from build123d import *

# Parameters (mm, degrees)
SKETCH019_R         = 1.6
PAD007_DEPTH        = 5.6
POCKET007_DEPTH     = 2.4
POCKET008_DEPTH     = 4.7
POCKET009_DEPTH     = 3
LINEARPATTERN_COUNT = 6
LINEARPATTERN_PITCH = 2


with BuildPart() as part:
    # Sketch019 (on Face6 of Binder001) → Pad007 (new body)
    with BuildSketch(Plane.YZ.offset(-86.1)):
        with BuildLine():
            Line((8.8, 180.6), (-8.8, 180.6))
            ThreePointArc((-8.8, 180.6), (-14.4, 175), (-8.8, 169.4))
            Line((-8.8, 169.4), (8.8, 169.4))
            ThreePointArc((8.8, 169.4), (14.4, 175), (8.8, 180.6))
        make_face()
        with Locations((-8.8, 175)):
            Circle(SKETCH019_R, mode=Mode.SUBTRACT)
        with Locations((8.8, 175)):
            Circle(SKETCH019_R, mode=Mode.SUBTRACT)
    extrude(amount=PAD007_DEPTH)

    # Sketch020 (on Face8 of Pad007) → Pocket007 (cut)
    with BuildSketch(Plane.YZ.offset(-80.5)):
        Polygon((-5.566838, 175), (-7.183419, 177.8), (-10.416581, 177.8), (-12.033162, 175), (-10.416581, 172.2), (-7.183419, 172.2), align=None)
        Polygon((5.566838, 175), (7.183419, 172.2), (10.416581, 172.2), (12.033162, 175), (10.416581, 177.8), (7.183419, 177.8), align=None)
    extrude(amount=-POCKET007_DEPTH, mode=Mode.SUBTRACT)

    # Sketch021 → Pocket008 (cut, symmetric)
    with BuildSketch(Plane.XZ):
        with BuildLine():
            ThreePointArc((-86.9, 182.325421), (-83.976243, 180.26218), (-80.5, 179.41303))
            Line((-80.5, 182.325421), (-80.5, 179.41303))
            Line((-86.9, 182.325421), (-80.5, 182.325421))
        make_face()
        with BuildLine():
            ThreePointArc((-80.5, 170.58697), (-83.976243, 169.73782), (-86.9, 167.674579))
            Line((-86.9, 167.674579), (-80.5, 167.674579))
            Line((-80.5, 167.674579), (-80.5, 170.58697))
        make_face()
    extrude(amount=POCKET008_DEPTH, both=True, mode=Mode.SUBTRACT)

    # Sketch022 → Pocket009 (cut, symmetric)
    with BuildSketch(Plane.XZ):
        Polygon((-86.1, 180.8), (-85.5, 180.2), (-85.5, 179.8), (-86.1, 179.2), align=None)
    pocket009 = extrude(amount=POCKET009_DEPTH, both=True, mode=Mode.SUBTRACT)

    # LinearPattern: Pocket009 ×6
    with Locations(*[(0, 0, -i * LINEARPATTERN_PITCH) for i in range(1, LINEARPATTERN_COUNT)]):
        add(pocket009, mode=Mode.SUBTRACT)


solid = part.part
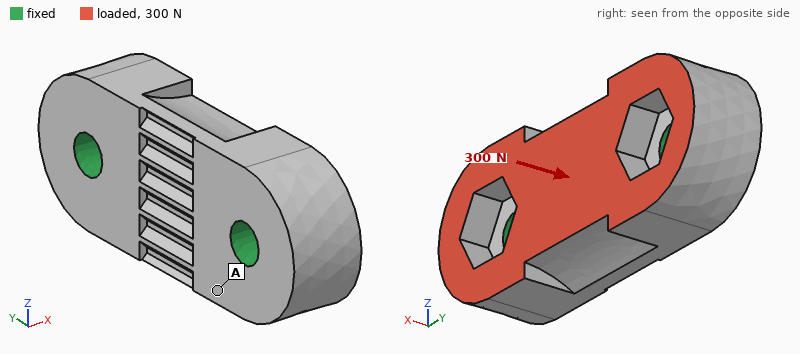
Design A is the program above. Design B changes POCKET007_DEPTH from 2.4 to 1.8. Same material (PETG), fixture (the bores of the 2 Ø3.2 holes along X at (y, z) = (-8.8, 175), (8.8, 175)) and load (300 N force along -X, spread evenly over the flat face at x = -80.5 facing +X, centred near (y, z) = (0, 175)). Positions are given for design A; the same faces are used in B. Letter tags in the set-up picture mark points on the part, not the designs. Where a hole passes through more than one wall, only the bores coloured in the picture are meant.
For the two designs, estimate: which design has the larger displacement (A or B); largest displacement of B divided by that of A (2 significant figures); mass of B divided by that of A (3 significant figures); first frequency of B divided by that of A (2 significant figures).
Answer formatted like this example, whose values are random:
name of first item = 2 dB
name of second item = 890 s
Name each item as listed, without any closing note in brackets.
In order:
which design has the larger displacement = A
largest displacement of B divided by that of A = 0.90
mass of B divided by that of A = 1.02
first frequency of B divided by that of A = 1.2
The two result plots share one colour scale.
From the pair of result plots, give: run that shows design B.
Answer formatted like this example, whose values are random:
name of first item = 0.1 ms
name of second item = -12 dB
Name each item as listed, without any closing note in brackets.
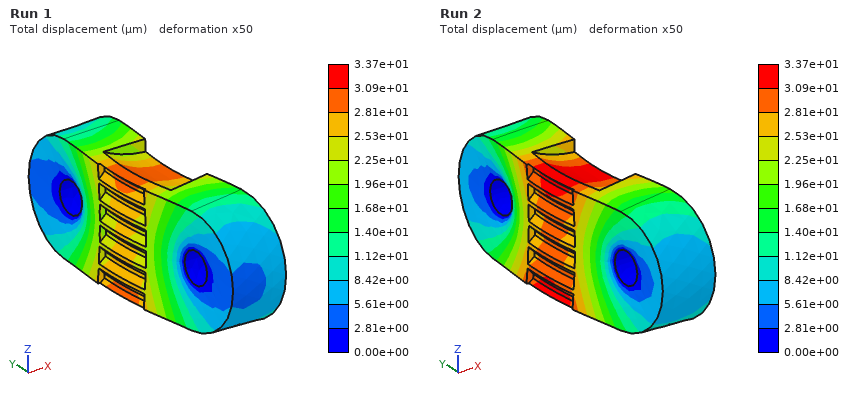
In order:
run that shows design B = Run 1
